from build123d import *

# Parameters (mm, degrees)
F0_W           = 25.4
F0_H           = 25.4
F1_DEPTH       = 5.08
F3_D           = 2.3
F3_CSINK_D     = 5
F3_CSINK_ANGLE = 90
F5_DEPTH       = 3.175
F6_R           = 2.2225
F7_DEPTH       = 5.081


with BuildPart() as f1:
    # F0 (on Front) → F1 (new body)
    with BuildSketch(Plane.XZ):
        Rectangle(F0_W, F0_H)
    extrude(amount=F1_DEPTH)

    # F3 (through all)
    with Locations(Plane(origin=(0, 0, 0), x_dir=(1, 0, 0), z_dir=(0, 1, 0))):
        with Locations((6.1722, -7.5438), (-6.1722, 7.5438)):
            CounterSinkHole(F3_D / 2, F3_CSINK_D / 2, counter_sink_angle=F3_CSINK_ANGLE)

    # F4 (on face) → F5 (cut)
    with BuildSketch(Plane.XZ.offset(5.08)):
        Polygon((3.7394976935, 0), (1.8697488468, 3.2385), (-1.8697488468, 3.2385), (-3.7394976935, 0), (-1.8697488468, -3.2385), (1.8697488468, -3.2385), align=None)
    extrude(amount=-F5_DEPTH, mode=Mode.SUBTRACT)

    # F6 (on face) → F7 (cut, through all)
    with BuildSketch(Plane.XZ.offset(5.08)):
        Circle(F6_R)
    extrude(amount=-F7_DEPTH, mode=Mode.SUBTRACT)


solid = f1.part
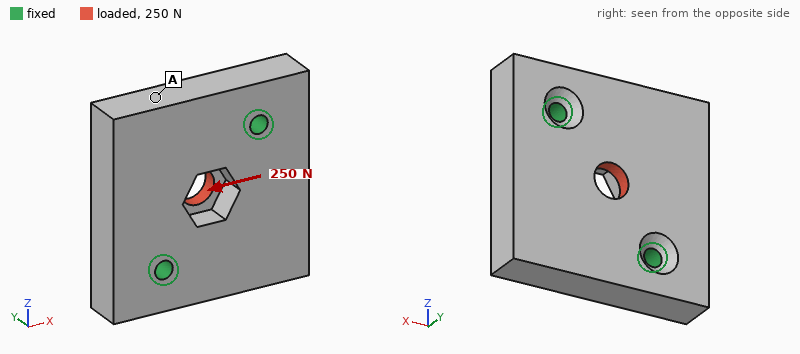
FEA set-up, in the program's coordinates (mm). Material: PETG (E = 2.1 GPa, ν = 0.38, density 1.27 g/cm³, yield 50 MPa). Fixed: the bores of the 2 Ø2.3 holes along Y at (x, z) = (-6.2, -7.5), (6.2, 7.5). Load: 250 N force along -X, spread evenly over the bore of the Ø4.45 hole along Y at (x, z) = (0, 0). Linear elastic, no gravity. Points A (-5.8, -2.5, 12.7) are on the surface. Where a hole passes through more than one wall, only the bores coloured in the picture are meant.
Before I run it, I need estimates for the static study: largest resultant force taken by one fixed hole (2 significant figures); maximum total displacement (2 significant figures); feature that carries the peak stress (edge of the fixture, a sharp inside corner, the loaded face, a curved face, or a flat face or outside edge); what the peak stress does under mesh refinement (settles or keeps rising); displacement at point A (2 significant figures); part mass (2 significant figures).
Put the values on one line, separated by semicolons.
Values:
130 N; 78 µm; edge of the fixture; keeps rising; 49 µm; 3.9 g
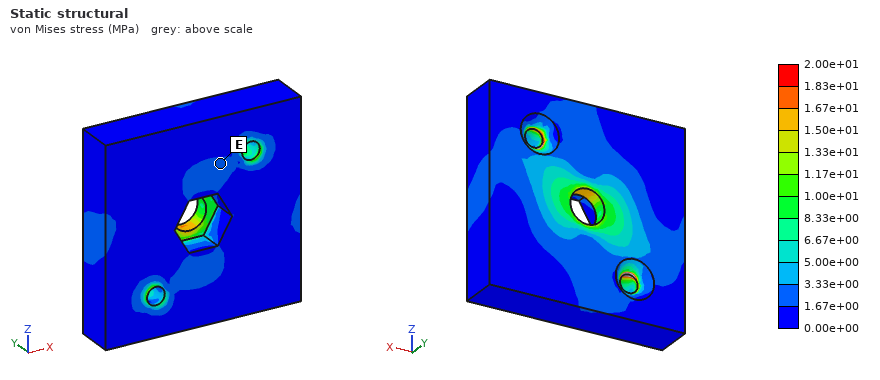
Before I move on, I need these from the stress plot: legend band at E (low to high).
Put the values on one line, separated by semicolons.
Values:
1.67e+00 to 3.33e+00 MPa
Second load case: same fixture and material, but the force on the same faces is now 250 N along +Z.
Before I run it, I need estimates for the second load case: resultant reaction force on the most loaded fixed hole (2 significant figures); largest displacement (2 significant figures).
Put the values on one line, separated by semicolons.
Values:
130 N; 67 µm
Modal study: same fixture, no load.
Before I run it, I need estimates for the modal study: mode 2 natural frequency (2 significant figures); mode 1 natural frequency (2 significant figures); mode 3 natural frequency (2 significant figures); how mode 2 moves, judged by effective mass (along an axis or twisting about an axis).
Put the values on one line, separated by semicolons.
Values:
4500 Hz; 3200 Hz; 10 kHz; along Y
